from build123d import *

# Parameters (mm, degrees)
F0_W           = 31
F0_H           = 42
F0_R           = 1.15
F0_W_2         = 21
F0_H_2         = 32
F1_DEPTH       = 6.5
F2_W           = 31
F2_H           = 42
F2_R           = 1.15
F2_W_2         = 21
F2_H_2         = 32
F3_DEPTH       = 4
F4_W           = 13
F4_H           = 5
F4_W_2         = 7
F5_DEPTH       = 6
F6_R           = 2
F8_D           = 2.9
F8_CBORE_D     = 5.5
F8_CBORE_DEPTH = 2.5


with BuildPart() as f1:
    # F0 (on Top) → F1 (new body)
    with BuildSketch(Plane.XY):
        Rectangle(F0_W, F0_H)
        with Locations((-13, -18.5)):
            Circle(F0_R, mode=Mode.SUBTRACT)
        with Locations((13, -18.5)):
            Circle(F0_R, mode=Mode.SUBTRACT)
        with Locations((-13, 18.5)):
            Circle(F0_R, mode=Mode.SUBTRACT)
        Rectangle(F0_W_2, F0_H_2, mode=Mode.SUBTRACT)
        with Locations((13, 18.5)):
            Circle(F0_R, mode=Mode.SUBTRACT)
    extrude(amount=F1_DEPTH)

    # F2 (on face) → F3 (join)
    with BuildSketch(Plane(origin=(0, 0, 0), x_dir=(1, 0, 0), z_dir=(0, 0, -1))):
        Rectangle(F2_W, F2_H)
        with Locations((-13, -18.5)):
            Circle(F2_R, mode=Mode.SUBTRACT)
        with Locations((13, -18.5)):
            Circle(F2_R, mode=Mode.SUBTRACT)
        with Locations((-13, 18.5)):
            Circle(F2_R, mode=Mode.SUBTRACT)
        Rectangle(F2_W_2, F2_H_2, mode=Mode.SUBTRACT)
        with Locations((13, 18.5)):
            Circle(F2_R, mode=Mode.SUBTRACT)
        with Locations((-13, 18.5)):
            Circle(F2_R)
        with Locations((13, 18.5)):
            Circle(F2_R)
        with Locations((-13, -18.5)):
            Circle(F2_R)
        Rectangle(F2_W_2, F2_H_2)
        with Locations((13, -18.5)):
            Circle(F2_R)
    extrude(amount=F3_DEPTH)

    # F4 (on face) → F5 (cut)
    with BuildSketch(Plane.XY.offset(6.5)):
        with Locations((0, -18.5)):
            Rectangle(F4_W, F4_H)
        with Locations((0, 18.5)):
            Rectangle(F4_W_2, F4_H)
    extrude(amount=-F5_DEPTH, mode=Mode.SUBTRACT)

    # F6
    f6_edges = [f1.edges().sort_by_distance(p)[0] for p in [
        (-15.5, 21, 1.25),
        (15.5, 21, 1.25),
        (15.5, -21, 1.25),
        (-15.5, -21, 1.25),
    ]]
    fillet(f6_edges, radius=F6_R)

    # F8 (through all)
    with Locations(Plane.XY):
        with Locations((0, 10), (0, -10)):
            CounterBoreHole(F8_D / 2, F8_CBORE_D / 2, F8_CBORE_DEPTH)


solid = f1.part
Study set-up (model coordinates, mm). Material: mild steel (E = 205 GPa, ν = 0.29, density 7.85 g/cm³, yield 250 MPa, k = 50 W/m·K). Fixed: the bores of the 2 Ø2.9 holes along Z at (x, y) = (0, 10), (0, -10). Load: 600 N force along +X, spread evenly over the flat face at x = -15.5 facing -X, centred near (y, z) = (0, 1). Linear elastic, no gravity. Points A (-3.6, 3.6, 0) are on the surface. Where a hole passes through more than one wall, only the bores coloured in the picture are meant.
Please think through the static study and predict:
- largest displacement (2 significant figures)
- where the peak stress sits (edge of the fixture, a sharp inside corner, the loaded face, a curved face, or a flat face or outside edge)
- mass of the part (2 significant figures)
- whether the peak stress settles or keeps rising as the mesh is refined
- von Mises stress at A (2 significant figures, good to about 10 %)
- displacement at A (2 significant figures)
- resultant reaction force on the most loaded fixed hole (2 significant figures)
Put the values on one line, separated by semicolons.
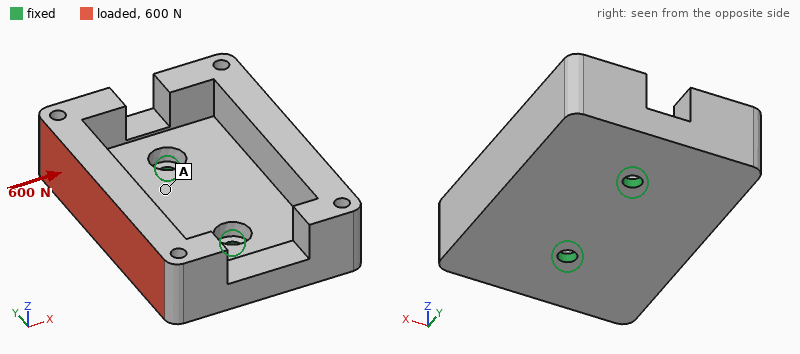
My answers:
24 µm; edge of the fixture; 66 g; keeps rising; 20 MPa; 5.5 µm; 300 N
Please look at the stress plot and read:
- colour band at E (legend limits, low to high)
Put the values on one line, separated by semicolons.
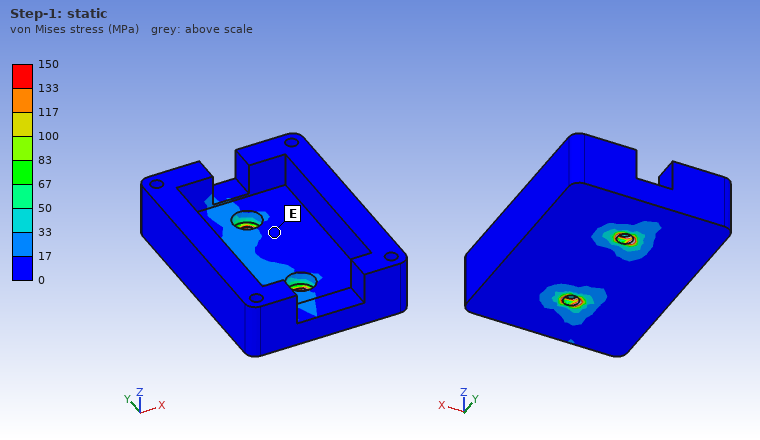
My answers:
0 to 17 MPa
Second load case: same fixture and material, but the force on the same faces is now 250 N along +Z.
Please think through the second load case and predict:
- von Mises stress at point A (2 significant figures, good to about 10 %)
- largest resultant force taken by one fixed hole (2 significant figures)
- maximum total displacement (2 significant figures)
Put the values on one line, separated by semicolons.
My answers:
26 MPa; 130 N; 33 µm
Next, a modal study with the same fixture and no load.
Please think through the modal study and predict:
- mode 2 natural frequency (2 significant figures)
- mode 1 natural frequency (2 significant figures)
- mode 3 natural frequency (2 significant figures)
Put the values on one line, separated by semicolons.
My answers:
8000 Hz; 2800 Hz; 8300 Hz
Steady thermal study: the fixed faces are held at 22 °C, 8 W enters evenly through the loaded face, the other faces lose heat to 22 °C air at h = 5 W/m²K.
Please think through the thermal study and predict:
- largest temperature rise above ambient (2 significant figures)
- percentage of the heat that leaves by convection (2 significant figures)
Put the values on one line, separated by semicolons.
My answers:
21 K; 3.1 %
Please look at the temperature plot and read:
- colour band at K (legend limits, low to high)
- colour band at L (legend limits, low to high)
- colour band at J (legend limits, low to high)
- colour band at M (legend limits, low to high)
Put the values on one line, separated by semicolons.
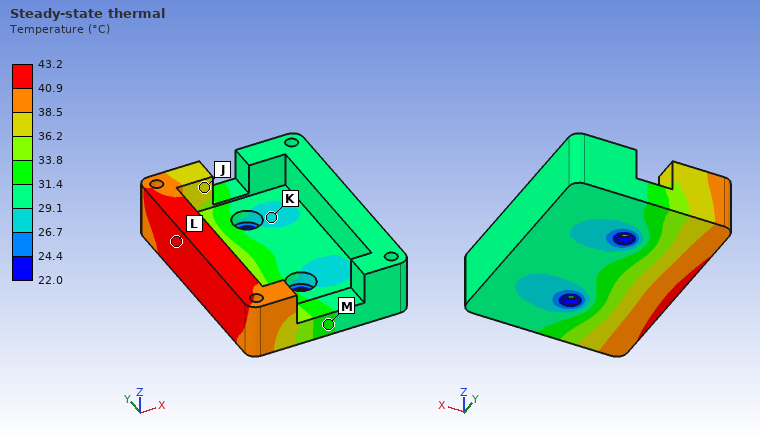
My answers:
26.7 to 29.1 °C; 40.9 to 43.2 °C; 36.2 to 38.5 °C; 31.4 to 33.8 °C
